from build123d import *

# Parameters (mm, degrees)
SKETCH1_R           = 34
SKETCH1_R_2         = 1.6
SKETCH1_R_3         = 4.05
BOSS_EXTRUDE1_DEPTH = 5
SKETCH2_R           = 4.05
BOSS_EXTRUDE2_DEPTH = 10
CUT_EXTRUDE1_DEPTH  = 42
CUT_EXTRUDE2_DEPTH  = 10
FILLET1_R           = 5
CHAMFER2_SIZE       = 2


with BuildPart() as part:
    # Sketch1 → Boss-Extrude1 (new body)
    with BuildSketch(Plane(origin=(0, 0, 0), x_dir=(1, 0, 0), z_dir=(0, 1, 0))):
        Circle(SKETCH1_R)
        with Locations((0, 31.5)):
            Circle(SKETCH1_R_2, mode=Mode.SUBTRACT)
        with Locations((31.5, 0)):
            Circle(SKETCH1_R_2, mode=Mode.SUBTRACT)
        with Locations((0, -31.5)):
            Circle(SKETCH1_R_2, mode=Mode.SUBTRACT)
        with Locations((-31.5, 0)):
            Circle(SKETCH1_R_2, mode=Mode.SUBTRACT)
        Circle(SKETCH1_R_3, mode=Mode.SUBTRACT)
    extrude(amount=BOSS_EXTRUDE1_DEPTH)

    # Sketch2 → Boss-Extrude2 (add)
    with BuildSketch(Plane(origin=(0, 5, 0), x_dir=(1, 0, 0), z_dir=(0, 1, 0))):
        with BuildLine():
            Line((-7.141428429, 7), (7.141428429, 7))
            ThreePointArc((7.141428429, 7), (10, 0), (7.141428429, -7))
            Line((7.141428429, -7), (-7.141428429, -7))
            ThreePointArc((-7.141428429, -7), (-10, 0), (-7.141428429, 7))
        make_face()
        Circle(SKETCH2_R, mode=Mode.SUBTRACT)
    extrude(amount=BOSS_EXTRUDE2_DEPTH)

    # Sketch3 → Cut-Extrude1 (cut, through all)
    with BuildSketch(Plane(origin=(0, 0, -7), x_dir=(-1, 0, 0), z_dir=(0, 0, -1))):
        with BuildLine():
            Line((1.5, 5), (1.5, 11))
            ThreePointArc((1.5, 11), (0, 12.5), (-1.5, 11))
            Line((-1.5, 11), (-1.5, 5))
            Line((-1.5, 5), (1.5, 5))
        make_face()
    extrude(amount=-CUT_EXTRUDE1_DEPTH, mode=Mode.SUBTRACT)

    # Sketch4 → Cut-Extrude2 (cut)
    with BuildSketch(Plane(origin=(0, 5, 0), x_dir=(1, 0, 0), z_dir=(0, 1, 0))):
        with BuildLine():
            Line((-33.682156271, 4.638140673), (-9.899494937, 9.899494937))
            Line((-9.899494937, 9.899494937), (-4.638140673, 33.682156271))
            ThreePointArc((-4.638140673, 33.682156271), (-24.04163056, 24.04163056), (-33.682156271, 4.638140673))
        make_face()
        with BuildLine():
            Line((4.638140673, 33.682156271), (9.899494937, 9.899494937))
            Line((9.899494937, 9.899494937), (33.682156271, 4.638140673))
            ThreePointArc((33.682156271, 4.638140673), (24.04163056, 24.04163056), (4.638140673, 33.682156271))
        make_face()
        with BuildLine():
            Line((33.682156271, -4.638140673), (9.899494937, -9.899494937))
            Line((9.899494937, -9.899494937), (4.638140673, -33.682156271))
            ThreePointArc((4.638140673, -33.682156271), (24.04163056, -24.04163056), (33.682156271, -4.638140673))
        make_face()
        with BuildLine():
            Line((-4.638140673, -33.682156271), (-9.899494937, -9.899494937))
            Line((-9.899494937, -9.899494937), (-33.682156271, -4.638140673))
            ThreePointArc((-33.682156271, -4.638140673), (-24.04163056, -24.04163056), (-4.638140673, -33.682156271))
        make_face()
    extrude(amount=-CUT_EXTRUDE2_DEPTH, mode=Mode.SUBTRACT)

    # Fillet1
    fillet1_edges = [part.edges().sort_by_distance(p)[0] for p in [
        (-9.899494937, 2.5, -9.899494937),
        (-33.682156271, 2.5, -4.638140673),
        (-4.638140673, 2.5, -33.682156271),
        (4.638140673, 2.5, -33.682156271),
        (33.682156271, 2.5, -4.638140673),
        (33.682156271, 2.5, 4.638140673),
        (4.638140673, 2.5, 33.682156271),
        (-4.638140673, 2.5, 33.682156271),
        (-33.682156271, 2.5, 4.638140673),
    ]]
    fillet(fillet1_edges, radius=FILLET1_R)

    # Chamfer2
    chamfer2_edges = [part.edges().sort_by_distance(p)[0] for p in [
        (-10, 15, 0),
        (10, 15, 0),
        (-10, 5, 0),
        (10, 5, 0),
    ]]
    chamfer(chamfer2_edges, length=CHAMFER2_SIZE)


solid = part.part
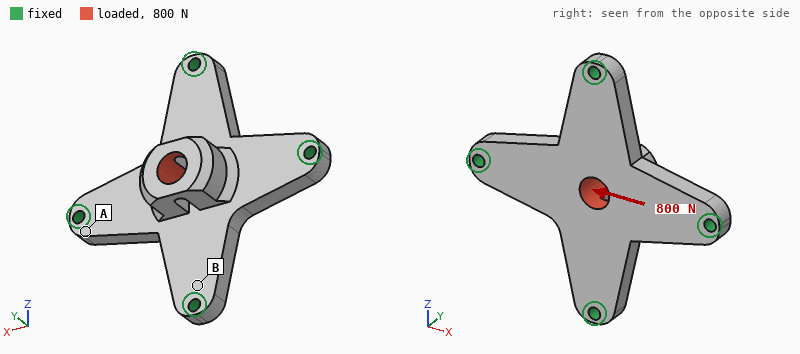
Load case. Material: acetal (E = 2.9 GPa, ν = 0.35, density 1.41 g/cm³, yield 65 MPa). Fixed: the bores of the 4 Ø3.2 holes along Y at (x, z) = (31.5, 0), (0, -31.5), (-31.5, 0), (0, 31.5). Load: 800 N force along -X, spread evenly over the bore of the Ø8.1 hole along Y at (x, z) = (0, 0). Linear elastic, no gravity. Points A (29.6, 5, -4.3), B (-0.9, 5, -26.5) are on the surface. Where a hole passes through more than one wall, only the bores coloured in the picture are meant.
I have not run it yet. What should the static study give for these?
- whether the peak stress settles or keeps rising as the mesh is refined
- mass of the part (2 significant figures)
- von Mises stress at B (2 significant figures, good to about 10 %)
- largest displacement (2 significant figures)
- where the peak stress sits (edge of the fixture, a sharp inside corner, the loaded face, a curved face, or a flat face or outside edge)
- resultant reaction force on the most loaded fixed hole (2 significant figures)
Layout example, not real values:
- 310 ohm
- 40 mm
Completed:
- keeps rising
- 15 g
- 5.2 MPa
- 0.19 mm
- edge of the fixture
- 370 N
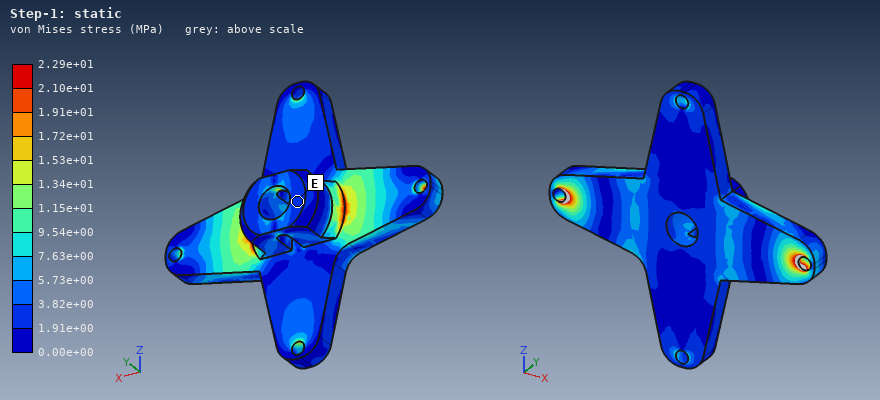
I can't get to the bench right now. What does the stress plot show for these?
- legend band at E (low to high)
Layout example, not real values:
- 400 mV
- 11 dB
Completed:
- 1.91e+00 to 3.82e+00 MPa
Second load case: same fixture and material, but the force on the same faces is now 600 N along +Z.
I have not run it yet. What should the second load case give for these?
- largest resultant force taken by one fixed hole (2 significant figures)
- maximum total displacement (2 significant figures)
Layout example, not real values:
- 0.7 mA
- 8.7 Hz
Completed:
- 280 N
- 0.20 mm
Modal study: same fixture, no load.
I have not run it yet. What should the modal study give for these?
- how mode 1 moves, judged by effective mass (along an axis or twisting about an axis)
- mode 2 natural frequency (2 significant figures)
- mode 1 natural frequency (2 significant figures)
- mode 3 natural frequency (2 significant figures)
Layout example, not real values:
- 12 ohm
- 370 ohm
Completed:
- along Y
- 3600 Hz
- 2000 Hz
- 3800 Hz
